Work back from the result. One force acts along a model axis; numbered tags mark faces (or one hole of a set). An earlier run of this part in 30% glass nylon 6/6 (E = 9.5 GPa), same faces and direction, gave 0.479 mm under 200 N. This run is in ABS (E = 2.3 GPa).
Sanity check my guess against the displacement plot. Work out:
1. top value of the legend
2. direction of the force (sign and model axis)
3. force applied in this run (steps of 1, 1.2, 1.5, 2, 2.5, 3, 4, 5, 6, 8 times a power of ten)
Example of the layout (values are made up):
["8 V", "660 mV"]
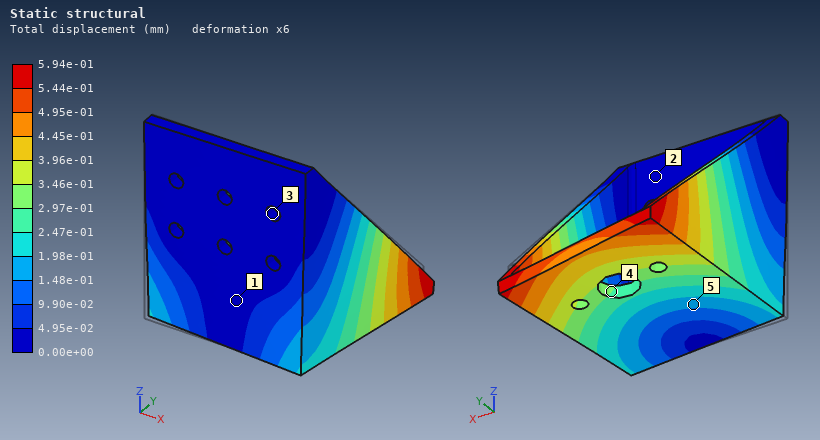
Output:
["5.94e-01 mm", "+X", "60 N"]
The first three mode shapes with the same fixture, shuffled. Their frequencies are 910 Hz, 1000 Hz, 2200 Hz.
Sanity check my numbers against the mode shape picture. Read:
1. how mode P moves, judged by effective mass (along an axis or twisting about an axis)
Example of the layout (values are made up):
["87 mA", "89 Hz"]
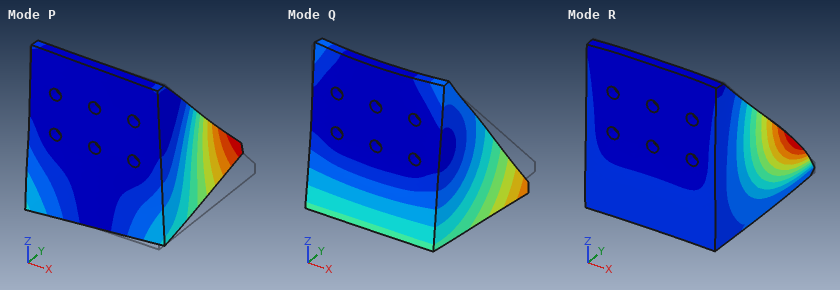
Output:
["along X"]
